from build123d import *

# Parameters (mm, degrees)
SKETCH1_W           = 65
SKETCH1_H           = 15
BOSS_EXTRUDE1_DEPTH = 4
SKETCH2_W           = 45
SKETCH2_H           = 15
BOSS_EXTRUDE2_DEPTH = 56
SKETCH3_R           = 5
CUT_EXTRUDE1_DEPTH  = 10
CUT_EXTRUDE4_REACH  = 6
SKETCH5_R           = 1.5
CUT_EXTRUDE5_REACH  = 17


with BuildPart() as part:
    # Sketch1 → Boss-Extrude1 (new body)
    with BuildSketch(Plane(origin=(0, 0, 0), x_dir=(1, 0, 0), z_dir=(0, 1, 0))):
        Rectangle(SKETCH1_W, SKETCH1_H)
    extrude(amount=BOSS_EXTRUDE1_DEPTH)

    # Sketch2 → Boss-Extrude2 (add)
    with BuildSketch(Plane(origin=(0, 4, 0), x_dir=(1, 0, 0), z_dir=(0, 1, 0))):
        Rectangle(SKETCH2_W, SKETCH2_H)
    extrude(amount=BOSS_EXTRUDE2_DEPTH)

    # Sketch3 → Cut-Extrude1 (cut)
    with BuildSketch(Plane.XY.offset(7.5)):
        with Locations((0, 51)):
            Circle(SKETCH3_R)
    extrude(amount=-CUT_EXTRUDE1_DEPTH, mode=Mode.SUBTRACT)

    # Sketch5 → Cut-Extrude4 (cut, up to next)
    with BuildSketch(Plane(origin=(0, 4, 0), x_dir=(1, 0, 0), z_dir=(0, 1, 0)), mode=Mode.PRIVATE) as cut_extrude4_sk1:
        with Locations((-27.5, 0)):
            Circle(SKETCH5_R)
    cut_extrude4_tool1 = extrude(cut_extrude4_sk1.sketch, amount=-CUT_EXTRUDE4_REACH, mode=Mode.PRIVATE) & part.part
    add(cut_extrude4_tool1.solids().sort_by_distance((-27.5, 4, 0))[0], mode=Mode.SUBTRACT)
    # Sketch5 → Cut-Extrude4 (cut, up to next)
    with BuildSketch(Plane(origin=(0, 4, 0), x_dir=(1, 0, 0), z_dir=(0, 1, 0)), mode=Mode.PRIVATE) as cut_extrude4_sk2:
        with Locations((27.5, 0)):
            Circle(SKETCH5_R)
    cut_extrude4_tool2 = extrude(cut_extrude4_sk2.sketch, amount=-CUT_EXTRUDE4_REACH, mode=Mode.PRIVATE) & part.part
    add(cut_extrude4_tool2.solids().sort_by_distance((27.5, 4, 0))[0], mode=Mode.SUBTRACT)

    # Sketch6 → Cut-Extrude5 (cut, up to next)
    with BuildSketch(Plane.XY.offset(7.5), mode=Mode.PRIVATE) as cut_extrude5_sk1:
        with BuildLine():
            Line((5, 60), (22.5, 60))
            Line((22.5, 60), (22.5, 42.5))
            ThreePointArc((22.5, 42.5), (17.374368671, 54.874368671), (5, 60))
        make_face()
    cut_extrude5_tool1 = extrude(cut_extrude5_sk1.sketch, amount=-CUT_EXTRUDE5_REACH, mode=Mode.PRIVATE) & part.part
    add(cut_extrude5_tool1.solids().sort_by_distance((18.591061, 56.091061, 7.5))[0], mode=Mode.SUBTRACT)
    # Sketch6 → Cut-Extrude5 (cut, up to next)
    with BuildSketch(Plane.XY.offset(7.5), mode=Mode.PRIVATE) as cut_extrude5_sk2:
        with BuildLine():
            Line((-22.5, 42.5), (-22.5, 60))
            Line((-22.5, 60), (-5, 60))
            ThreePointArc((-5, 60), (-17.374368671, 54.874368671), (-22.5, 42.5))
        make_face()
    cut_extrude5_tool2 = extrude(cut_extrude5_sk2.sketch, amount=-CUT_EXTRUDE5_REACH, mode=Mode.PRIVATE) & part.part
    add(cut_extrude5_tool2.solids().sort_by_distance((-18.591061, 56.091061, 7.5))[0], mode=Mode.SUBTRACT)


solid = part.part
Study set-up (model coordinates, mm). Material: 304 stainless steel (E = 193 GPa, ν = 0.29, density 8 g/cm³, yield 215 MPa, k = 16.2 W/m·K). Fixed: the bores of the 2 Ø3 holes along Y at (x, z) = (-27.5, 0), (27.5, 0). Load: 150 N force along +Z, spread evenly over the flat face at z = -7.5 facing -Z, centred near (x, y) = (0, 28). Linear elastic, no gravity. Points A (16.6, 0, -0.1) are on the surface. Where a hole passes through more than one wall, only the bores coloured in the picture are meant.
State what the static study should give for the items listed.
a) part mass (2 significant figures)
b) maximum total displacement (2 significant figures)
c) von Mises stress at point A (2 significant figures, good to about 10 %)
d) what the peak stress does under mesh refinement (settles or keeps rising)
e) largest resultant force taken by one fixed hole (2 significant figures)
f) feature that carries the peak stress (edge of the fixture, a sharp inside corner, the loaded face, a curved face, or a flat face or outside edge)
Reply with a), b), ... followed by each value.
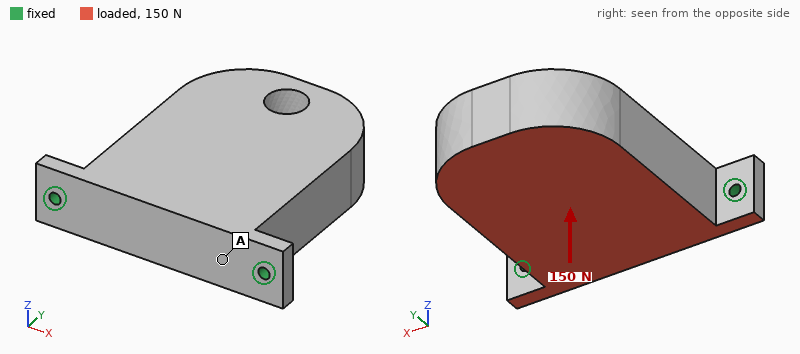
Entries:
a) 310 g
b) 33 µm
c) 5.4 MPa
d) keeps rising
e) 75 N
f) edge of the fixture
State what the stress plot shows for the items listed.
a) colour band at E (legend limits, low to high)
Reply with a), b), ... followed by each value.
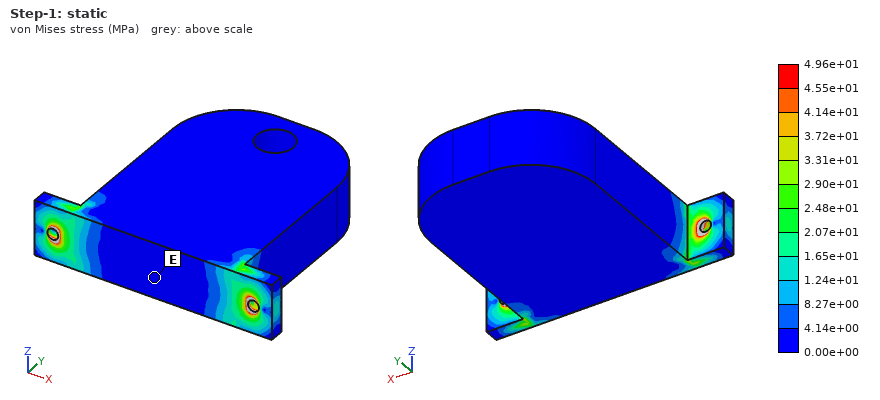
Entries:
a) 0.00e+00 to 4.14e+00 MPa
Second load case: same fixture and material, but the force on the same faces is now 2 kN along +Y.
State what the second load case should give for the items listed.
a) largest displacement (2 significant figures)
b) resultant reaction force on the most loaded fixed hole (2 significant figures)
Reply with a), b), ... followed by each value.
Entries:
a) 0.13 mm
b) 1.1 kN
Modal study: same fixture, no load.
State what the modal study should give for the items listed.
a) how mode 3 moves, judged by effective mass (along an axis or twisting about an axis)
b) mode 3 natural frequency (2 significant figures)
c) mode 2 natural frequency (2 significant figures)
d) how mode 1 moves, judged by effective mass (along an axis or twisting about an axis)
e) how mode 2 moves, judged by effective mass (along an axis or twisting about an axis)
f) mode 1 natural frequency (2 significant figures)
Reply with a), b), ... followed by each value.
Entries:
a) along Y
b) 5700 Hz
c) 4000 Hz
d) along Z
e) along X
f) 770 Hz
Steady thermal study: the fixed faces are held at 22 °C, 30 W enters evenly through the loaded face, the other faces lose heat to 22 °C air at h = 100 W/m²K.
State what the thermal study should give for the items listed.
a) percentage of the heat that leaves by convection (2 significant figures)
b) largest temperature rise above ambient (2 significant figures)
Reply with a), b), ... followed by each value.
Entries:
a) 77 %
b) 51 K
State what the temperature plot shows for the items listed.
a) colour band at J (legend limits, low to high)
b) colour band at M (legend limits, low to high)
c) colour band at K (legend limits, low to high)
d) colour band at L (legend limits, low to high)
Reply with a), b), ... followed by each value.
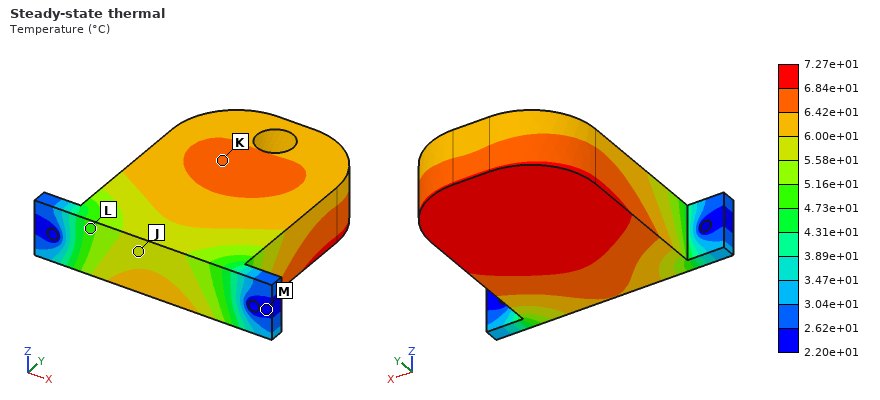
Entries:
a) 5.58e+01 to 6.00e+01 °C
b) 2.20e+01 to 2.62e+01 °C
c) 6.42e+01 to 6.84e+01 °C
d) 4.73e+01 to 5.16e+01 °C
